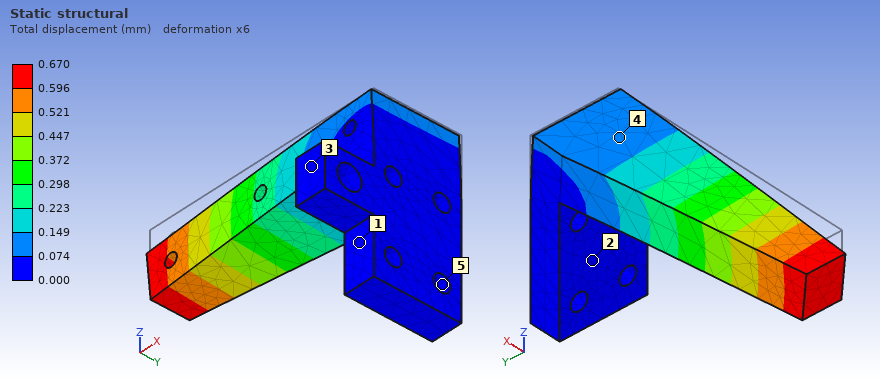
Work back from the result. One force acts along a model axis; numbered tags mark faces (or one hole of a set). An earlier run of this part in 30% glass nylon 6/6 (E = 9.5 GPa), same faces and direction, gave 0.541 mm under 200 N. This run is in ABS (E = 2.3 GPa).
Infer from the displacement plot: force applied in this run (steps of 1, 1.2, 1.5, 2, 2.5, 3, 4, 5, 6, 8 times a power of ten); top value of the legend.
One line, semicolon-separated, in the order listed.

60 N; 0.670 mm
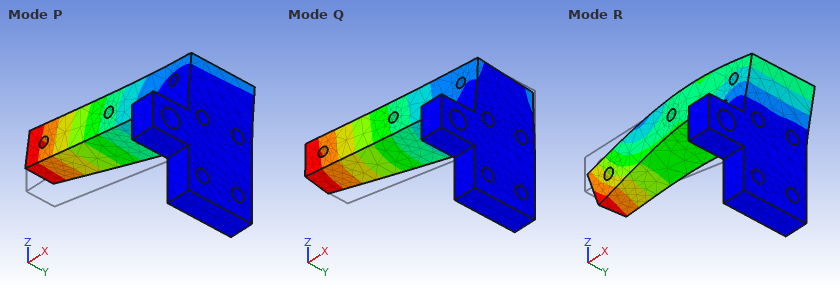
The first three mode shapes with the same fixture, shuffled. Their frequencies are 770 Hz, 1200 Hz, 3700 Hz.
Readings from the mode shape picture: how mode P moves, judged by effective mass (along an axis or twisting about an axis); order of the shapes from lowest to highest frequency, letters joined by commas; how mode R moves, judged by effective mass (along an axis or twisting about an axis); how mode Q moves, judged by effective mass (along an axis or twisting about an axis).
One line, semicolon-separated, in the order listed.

along Z; P, Q, R; along X; along Y
